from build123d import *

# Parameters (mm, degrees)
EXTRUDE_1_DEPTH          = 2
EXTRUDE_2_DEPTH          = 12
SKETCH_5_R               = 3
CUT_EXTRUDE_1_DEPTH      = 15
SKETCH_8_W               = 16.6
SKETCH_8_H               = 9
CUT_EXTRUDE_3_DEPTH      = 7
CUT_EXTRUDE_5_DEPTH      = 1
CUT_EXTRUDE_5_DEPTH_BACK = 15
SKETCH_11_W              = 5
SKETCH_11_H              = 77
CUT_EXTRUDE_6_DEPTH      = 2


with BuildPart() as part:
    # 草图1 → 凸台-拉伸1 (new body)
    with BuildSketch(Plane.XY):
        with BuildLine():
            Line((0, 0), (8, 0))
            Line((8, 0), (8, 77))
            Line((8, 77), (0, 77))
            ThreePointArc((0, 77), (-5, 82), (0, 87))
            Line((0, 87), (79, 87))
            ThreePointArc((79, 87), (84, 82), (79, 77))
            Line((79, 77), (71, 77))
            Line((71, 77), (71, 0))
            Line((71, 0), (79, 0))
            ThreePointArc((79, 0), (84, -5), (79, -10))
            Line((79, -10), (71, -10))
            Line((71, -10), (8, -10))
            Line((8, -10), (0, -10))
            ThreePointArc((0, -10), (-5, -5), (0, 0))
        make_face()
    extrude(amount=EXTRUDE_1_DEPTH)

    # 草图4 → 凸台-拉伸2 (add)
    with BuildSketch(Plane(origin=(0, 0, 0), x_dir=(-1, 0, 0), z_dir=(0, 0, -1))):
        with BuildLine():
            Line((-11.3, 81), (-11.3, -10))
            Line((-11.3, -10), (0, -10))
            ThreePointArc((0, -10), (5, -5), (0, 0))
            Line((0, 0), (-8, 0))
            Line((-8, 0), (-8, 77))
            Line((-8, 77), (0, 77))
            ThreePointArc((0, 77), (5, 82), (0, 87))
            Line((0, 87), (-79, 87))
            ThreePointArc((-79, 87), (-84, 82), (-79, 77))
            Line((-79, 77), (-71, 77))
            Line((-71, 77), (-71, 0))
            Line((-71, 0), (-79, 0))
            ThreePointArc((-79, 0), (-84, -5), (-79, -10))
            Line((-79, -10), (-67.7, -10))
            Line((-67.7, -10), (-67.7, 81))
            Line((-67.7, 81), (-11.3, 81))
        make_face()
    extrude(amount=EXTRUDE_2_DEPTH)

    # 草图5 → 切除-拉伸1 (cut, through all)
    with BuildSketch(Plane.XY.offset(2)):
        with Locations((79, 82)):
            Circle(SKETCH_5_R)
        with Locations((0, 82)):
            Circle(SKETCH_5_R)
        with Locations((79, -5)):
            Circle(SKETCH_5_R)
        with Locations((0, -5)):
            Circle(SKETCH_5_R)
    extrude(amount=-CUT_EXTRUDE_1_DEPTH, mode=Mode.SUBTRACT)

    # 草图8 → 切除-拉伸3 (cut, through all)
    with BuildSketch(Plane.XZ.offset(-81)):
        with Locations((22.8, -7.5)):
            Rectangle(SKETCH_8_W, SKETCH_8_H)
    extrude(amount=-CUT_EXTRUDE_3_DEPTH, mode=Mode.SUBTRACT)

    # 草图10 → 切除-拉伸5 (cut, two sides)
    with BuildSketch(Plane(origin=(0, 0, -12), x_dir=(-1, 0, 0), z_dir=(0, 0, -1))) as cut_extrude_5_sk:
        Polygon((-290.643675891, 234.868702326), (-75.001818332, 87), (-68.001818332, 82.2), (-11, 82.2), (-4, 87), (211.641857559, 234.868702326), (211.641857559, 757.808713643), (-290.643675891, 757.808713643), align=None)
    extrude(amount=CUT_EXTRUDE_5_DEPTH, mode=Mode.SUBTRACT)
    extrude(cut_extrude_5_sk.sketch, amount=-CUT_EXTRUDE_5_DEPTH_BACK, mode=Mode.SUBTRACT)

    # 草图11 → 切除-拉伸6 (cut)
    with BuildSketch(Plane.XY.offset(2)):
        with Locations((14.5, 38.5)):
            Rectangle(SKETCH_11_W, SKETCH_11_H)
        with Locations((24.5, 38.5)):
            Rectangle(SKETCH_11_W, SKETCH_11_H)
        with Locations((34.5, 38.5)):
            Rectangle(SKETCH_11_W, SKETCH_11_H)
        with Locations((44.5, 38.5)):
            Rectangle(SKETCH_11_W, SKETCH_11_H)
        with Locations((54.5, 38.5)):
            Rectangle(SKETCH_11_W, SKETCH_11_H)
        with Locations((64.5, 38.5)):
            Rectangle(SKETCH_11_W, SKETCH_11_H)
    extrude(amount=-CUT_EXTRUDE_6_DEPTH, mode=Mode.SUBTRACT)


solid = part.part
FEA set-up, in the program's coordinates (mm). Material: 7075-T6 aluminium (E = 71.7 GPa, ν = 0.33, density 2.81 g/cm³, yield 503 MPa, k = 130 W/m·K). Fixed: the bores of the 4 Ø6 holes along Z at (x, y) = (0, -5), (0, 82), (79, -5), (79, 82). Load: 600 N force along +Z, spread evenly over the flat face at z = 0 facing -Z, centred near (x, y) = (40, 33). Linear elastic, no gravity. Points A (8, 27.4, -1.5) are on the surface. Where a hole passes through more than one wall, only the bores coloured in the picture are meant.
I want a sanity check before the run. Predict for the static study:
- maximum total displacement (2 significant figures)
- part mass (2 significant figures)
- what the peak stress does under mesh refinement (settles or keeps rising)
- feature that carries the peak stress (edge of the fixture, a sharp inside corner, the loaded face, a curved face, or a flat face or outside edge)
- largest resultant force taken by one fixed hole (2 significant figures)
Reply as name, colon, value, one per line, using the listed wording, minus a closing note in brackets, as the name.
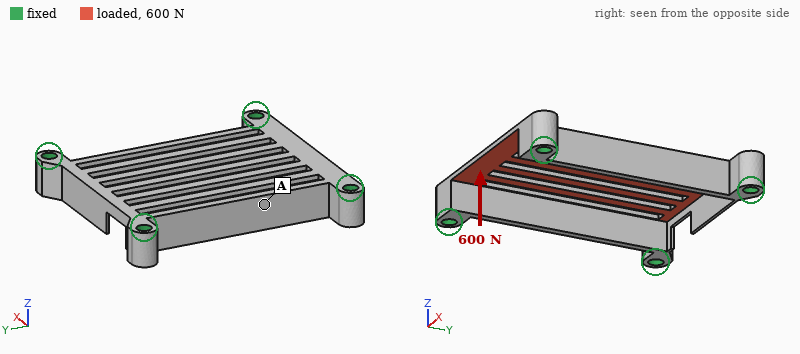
maximum total displacement: 1.5 mm
part mass: 56 g
what the peak stress does under mesh refinement: keeps rising
feature that carries the peak stress: a sharp inside corner
largest resultant force taken by one fixed hole: 190 N
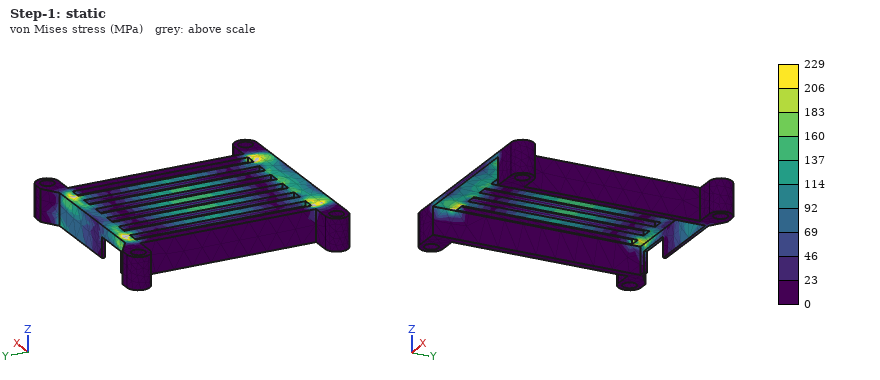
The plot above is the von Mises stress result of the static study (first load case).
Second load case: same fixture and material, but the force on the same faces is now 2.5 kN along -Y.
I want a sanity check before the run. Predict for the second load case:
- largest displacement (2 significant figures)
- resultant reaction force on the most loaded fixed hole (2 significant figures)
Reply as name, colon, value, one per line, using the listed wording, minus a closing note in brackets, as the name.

largest displacement: 0.16 mm
resultant reaction force on the most loaded fixed hole: 730 N
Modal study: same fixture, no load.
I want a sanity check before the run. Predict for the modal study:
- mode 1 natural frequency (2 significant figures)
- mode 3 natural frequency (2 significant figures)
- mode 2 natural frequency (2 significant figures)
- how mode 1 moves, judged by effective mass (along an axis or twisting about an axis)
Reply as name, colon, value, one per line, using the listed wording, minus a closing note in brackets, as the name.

mode 1 natural frequency: 990 Hz
mode 3 natural frequency: 1400 Hz
mode 2 natural frequency: 1300 Hz
how mode 1 moves, judged by effective mass: along Z
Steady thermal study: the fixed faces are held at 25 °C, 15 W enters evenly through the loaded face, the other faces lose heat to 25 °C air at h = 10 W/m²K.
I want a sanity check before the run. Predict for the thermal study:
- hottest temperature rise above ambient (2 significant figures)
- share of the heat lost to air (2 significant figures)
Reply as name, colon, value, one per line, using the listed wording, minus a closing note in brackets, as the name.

hottest temperature rise above ambient: 37 K
share of the heat lost to air: 9.7 %
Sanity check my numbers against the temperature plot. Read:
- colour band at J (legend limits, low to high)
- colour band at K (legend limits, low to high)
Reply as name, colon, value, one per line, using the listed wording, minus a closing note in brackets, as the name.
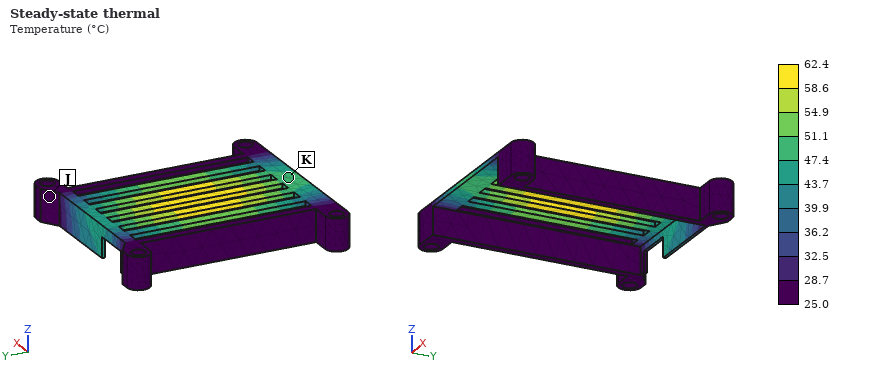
colour band at J: 25.0 to 28.7 °C
colour band at K: 47.4 to 51.1 °C
